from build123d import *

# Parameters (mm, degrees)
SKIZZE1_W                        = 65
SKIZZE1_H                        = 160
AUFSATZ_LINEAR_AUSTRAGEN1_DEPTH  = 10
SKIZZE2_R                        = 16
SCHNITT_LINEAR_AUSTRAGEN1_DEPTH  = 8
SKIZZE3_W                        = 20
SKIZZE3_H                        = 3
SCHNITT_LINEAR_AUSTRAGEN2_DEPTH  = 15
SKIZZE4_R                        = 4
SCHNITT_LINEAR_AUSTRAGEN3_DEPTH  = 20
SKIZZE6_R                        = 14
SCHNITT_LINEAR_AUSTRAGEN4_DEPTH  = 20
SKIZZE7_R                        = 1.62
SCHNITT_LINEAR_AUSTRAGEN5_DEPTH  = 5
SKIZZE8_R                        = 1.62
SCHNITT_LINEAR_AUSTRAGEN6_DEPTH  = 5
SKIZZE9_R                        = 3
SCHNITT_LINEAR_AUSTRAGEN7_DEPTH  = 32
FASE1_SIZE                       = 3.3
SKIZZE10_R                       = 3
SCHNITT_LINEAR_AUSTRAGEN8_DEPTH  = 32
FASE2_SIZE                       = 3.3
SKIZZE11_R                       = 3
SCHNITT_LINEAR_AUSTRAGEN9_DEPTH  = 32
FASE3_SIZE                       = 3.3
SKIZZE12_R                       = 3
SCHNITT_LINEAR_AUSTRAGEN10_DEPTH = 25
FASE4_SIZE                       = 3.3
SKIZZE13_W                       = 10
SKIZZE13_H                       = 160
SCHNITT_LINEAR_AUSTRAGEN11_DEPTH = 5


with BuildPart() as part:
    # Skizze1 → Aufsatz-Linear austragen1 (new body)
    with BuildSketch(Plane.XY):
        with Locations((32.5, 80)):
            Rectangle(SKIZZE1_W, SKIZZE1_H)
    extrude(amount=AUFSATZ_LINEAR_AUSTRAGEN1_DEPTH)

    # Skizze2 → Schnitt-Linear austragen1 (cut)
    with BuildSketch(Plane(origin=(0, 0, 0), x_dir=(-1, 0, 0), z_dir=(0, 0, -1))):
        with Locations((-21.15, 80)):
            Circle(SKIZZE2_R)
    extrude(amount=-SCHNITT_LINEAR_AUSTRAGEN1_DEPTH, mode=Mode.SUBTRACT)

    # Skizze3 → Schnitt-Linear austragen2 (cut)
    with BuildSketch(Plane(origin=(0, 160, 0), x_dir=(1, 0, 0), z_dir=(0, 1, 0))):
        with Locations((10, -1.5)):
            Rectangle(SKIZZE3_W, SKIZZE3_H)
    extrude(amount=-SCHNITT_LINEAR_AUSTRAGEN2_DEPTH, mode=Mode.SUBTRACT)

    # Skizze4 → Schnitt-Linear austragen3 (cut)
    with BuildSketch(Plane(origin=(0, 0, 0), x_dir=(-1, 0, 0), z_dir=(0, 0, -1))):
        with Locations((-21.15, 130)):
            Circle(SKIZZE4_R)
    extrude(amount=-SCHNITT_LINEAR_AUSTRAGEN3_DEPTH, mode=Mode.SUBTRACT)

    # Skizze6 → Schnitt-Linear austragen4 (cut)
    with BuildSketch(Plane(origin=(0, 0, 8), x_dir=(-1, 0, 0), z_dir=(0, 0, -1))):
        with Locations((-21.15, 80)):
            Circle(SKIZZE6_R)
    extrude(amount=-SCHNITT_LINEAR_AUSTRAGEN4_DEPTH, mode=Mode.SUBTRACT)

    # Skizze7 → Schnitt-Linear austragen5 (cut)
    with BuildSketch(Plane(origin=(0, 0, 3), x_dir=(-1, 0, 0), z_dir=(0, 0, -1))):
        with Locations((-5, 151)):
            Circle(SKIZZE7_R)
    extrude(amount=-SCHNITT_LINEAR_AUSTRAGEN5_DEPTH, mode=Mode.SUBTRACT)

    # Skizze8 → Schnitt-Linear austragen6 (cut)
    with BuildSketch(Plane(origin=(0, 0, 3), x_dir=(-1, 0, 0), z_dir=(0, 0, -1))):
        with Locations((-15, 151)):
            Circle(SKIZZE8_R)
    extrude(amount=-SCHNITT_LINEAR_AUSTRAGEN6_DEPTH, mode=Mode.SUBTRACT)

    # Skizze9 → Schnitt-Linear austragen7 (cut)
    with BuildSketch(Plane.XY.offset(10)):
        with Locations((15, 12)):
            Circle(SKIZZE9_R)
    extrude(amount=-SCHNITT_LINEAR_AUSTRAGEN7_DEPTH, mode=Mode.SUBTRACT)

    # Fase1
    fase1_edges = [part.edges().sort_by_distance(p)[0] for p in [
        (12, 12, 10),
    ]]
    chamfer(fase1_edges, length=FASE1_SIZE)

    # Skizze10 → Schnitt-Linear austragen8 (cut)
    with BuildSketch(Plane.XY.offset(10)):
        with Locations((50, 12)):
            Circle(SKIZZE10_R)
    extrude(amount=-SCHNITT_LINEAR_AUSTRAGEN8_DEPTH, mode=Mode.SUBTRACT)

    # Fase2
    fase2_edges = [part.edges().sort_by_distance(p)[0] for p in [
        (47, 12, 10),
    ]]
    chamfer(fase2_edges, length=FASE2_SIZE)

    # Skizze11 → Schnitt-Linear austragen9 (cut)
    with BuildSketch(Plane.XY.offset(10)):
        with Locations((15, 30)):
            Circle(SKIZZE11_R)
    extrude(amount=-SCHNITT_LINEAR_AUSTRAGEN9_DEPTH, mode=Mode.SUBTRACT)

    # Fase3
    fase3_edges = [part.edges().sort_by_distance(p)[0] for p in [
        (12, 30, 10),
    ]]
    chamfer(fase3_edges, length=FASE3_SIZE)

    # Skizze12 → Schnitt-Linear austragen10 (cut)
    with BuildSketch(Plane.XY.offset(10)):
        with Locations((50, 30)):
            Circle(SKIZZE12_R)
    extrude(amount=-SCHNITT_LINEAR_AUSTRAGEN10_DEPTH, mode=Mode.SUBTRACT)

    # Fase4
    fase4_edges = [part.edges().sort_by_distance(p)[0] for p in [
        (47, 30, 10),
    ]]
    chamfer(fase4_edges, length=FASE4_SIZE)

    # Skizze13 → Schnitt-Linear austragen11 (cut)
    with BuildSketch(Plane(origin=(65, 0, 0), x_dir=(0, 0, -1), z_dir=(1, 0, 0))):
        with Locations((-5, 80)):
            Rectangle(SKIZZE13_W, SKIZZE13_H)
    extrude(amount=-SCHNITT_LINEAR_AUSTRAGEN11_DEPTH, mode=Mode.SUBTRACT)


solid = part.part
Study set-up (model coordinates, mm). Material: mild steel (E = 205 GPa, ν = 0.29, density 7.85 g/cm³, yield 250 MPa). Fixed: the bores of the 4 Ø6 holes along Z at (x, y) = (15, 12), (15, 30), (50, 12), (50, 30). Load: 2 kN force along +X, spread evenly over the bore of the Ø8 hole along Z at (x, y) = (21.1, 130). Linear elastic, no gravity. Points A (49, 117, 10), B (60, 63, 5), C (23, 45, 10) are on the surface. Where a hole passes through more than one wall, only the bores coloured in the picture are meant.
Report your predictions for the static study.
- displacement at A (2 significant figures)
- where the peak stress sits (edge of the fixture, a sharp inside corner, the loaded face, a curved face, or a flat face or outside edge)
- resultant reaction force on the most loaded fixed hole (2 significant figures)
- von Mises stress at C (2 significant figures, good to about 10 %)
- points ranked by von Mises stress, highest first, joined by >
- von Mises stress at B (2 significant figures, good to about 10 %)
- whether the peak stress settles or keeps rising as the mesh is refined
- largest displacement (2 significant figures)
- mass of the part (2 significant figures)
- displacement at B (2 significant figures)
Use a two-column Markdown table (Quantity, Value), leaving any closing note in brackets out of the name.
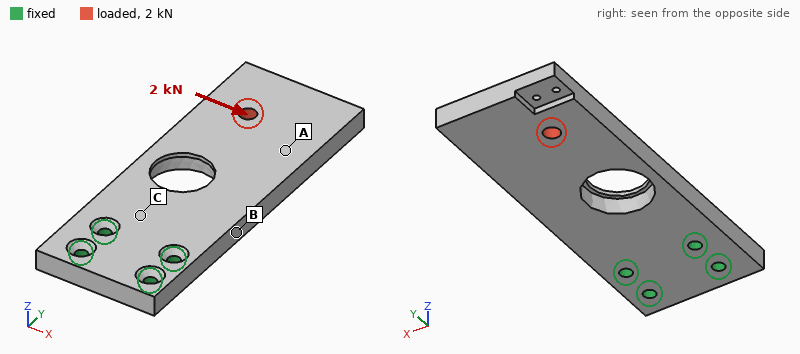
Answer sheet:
| Quantity | Value |
|---|---|
| displacement at A | 31 µm |
| where the peak stress sits | edge of the fixture |
| resultant reaction force on the most loaded fixed hole | 4.2 kN |
| von Mises stress at C | 14 MPa |
| points ranked by von Mises stress, highest first, joined by > | B > C > A |
| von Mises stress at B | 35 MPa |
| whether the peak stress settles or keeps rising as the mesh is refined | keeps rising |
| largest displacement | 50 µm |
| mass of the part | 670 g |
| displacement at B | 9.3 µm |
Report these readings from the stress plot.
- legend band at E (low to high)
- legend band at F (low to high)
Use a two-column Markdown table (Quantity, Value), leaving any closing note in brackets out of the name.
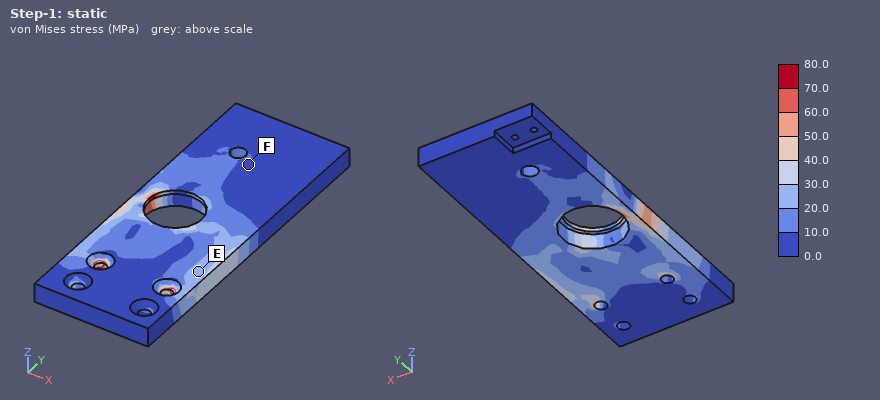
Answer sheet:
| Quantity | Value |
|---|---|
| legend band at E | 20.0 to 30.0 MPa |
| legend band at F | 0.0 to 10.0 MPa |
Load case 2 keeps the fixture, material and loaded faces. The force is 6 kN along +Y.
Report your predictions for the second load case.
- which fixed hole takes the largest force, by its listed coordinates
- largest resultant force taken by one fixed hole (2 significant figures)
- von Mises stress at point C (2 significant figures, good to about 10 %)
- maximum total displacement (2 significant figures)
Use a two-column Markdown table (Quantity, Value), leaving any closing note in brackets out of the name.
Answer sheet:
| Quantity | Value |
|---|---|
| which fixed hole takes the largest force, by its listed coordinates | (15, 30) |
| largest resultant force taken by one fixed hole | 3.4 kN |
| von Mises stress at point C | 7.0 MPa |
| maximum total displacement | 31 µm |
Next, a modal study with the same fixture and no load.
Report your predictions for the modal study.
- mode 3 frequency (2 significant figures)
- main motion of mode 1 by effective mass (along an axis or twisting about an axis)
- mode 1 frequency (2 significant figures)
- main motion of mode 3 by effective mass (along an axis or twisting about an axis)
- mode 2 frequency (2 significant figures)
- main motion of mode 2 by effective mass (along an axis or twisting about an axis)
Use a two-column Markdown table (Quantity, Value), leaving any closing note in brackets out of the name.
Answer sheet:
| Quantity | Value |
|---|---|
| mode 3 frequency | 2100 Hz |
| main motion of mode 1 by effective mass | along Z |
| mode 1 frequency | 430 Hz |
| main motion of mode 3 by effective mass | along X |
| mode 2 frequency | 1900 Hz |
| main motion of mode 2 by effective mass | twisting about Y |
